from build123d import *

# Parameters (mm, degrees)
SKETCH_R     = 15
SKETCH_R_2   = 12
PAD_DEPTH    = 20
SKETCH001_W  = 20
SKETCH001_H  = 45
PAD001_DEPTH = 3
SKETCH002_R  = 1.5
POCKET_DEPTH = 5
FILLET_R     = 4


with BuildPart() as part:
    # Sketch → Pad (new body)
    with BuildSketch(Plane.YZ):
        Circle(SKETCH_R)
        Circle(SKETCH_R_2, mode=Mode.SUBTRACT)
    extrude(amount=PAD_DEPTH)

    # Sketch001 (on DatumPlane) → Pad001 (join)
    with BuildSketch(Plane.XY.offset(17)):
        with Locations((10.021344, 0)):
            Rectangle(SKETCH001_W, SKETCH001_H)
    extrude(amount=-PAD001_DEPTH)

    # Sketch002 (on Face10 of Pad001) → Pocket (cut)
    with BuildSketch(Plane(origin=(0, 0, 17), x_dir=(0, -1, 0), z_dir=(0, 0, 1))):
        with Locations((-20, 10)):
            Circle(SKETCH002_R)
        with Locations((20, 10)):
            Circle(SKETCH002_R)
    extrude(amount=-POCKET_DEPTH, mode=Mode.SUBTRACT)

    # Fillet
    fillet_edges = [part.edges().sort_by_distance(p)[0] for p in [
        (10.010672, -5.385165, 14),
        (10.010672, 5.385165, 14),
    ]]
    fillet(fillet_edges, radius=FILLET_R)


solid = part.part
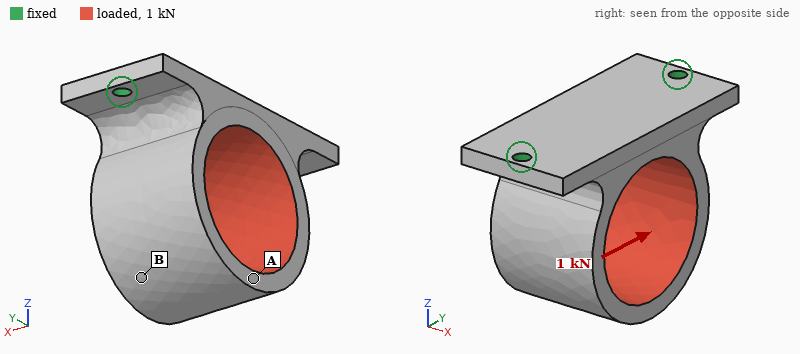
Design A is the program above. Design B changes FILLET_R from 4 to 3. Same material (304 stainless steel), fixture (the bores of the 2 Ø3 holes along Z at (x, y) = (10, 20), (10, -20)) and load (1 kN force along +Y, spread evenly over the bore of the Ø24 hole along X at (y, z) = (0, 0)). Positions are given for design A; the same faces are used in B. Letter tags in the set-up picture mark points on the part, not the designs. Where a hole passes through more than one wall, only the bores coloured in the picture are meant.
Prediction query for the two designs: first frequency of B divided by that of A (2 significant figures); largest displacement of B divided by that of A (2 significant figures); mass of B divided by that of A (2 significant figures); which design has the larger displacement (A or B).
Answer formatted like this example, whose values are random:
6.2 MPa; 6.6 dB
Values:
0.93; 1.3; 0.97; B
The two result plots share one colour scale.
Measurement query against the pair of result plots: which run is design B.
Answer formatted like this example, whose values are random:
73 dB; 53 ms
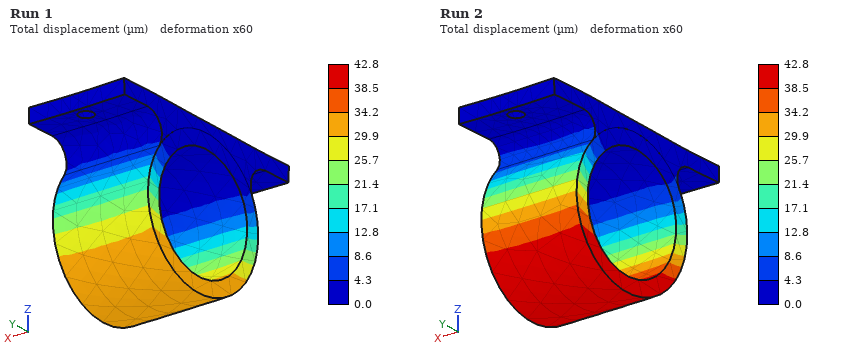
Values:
Run 2
